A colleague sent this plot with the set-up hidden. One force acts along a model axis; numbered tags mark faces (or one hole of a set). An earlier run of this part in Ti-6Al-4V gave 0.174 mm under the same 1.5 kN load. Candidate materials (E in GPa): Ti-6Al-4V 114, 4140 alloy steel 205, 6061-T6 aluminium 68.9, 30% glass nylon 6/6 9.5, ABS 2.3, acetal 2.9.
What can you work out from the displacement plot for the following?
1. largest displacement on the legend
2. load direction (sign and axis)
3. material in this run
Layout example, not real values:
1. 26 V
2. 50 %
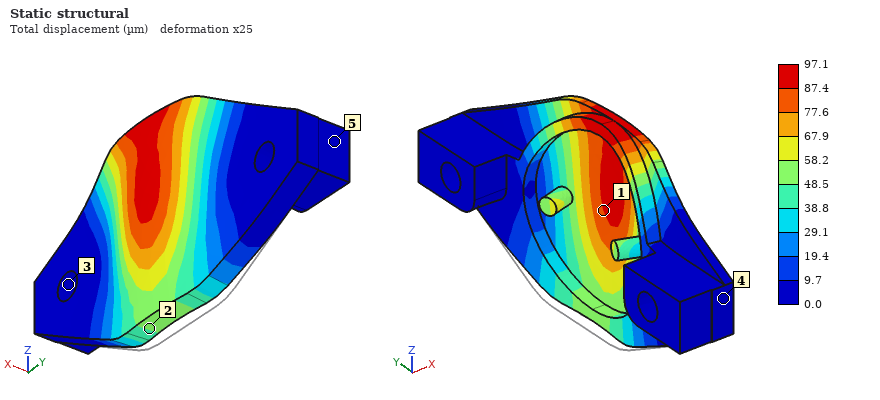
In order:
1. 97.1 µm
2. +X
3. 4140 alloy steel
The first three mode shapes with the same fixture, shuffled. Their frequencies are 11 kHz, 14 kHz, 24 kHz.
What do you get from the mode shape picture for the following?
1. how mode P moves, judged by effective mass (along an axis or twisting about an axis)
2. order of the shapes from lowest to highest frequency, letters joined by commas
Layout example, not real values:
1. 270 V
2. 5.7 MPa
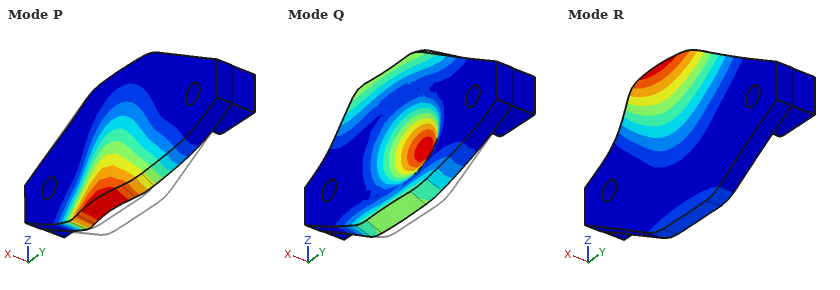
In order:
1. along X
2. R, P, Q
